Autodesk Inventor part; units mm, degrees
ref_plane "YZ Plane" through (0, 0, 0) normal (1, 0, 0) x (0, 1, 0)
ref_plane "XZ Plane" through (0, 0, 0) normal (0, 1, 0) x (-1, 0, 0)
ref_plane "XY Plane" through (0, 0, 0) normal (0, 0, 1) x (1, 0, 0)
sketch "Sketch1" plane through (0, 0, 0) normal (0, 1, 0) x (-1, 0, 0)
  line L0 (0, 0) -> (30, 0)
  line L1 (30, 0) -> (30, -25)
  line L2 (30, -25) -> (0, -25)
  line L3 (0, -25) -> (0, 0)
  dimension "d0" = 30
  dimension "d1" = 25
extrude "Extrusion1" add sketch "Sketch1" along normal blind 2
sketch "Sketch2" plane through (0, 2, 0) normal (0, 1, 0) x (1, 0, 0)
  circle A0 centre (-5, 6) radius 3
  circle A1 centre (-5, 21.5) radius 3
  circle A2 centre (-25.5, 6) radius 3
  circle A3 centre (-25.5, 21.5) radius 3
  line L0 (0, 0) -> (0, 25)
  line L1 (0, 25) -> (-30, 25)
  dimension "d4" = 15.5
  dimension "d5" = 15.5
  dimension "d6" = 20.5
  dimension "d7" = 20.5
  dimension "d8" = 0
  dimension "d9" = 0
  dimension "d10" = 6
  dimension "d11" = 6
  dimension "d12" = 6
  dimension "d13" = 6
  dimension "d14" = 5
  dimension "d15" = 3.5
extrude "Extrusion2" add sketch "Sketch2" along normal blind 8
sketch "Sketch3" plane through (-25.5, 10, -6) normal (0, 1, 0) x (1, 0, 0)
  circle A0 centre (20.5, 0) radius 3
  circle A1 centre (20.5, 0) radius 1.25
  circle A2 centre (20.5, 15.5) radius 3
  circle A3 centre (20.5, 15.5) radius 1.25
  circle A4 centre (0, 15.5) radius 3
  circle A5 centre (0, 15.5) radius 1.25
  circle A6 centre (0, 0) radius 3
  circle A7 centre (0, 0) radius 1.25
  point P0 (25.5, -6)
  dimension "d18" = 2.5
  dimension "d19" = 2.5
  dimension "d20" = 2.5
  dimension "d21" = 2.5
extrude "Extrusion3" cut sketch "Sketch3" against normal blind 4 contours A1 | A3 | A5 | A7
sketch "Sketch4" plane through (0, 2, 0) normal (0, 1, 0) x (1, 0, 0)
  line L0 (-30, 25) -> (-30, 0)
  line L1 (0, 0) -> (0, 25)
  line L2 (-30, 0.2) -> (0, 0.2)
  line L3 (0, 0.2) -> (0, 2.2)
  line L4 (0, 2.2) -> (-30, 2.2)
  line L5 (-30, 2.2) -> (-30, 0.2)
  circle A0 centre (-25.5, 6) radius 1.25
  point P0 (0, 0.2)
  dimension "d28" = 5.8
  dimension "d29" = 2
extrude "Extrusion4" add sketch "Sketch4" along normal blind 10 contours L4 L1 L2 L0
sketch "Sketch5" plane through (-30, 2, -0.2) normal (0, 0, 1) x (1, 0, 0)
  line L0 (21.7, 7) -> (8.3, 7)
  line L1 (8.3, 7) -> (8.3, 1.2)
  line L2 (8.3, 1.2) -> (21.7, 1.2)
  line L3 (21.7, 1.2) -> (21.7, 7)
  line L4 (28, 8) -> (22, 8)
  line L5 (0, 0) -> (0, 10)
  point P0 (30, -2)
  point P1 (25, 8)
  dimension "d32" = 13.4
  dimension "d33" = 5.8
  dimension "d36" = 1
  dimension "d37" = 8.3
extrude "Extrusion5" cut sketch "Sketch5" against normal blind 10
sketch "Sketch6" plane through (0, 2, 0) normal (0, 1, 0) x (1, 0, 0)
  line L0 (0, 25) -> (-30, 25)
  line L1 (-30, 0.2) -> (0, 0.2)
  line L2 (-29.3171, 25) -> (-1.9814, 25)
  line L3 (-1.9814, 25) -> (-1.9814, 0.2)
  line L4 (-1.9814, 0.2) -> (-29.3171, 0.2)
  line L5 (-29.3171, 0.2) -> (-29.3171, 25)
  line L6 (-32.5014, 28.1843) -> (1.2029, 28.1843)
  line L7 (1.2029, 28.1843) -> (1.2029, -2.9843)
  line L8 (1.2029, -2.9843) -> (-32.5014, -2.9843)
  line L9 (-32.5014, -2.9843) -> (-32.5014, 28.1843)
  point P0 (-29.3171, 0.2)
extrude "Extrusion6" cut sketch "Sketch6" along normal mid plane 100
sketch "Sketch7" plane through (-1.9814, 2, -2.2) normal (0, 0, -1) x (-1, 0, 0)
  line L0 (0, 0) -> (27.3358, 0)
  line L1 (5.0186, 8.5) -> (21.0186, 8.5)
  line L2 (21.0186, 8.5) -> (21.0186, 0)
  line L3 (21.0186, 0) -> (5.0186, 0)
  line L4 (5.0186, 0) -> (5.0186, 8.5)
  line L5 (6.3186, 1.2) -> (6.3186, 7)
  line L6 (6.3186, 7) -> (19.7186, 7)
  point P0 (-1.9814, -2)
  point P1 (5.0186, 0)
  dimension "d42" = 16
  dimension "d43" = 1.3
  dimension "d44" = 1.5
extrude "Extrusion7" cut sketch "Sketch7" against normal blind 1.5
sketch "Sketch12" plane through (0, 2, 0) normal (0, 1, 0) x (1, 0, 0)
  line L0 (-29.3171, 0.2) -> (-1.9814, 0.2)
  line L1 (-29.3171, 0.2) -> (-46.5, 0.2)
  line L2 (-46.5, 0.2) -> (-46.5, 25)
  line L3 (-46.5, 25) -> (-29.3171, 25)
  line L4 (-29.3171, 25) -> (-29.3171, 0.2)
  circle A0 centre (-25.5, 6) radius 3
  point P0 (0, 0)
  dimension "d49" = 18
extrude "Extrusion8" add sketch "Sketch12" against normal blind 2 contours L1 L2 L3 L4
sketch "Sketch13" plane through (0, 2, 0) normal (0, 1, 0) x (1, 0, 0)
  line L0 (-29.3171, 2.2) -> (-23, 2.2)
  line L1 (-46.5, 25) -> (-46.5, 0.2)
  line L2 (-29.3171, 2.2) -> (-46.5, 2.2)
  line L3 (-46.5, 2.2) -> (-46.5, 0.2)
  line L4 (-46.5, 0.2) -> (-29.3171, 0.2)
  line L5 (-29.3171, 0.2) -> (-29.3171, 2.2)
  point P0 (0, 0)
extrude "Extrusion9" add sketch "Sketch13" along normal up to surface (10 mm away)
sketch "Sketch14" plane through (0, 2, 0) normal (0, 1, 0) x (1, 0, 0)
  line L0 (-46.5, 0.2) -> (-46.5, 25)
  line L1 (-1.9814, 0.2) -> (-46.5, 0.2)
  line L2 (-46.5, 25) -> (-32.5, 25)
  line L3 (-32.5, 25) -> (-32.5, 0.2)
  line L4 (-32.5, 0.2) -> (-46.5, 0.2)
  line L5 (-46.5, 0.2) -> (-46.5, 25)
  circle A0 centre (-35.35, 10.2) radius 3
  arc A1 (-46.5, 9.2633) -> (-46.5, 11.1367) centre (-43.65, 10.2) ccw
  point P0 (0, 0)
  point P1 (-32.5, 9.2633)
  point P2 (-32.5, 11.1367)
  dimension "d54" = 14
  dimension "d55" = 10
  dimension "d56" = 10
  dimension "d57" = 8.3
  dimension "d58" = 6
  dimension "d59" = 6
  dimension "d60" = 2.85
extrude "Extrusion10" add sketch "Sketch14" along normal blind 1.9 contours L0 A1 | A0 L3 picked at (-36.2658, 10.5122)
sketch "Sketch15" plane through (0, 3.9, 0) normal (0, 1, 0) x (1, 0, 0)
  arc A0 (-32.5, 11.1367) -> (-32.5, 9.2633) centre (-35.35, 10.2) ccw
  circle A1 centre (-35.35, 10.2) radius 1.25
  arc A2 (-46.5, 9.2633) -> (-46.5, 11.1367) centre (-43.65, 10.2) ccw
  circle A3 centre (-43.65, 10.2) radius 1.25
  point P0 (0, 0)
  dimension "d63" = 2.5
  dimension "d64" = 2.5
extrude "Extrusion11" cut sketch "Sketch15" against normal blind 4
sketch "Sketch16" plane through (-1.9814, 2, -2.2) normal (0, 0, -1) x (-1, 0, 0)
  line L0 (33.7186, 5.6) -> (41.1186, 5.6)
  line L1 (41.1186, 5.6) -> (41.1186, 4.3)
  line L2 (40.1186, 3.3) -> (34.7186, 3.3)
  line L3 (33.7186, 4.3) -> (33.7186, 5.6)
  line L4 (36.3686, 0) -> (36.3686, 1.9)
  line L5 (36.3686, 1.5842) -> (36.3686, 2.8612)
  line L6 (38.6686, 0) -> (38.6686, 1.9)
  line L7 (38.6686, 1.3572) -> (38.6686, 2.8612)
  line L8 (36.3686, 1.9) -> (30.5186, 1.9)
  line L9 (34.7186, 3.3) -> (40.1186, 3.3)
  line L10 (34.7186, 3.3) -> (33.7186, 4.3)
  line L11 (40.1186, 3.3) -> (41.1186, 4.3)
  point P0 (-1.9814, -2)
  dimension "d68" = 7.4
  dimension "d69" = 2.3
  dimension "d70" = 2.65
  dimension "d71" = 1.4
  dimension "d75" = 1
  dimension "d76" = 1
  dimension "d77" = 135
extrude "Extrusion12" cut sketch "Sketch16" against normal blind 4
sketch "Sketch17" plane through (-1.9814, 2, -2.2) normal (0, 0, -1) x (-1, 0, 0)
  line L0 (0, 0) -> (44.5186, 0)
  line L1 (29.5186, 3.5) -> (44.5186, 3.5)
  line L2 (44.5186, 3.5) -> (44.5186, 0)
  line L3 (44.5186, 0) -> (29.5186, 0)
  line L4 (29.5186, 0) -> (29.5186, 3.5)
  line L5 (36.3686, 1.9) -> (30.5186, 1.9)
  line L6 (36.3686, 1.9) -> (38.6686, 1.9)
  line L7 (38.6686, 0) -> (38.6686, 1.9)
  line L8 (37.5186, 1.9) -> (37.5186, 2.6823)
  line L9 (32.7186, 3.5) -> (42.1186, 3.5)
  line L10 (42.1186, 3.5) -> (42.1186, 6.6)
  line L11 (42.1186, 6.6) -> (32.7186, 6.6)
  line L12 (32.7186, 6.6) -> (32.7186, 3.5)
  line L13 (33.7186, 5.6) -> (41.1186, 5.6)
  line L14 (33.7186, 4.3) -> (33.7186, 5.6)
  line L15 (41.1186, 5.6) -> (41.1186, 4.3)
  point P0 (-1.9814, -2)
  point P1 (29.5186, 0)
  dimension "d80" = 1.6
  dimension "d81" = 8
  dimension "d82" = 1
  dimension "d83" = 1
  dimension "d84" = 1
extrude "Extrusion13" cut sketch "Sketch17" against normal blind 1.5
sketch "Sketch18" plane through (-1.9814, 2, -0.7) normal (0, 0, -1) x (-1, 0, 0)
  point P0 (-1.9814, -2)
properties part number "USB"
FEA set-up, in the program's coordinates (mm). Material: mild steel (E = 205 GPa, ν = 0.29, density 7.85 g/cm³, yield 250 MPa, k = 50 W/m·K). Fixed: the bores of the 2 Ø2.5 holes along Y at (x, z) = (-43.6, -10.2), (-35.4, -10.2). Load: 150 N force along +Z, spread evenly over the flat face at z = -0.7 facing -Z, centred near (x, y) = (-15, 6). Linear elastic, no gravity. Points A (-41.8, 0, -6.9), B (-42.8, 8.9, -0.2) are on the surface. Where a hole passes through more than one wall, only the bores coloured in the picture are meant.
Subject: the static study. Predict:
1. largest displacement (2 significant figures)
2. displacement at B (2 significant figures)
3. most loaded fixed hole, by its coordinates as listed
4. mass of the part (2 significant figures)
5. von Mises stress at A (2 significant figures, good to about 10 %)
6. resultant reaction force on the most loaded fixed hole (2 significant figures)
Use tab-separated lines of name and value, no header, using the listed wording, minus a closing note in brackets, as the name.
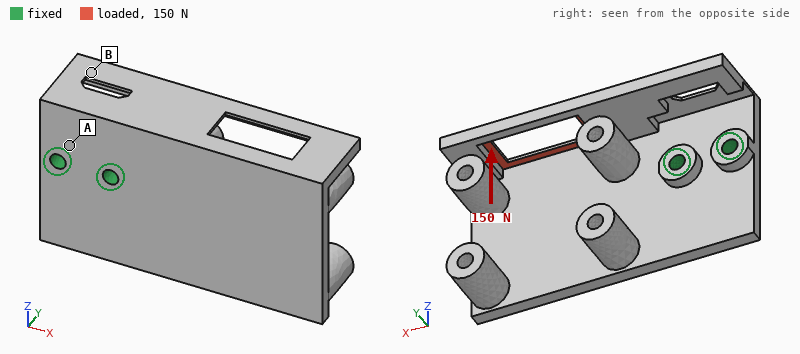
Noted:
largest displacement	64 µm
displacement at B	10 µm
most loaded fixed hole, by its coordinates as listed	(-35.4, -10.2)
mass of the part	28 g
von Mises stress at A	30 MPa
resultant reaction force on the most loaded fixed hole	420 N
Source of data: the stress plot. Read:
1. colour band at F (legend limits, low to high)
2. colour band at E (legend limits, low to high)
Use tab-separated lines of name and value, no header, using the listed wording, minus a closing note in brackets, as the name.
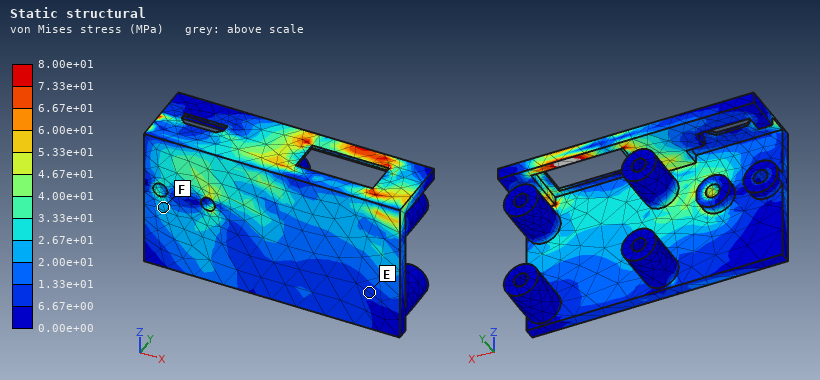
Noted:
colour band at F	2.00e+01 to 2.67e+01 MPa
colour band at E	6.67e+00 to 1.33e+01 MPa
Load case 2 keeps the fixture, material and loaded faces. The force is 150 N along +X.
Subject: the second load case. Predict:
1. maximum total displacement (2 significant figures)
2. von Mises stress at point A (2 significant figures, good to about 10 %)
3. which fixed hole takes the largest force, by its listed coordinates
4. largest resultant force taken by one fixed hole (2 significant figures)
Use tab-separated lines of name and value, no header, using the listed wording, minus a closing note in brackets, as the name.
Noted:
maximum total displacement	35 µm
von Mises stress at point A	24 MPa
which fixed hole takes the largest force, by its listed coordinates	(-35.4, -10.2)
largest resultant force taken by one fixed hole	180 N
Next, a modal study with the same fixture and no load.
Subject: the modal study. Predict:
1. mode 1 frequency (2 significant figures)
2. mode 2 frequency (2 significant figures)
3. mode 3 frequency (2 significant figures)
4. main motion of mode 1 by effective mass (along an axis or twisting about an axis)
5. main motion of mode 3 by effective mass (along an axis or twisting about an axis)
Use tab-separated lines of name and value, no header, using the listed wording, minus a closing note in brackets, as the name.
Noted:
mode 1 frequency	1500 Hz
mode 2 frequency	2500 Hz
mode 3 frequency	5800 Hz
main motion of mode 1 by effective mass	along Y
main motion of mode 3 by effective mass	along Z
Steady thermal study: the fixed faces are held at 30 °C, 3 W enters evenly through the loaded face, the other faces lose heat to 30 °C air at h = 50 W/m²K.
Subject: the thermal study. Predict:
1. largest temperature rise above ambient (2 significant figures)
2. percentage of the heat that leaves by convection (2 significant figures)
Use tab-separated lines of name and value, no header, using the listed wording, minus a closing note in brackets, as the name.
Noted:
largest temperature rise above ambient	36 K
percentage of the heat that leaves by convection	54 %
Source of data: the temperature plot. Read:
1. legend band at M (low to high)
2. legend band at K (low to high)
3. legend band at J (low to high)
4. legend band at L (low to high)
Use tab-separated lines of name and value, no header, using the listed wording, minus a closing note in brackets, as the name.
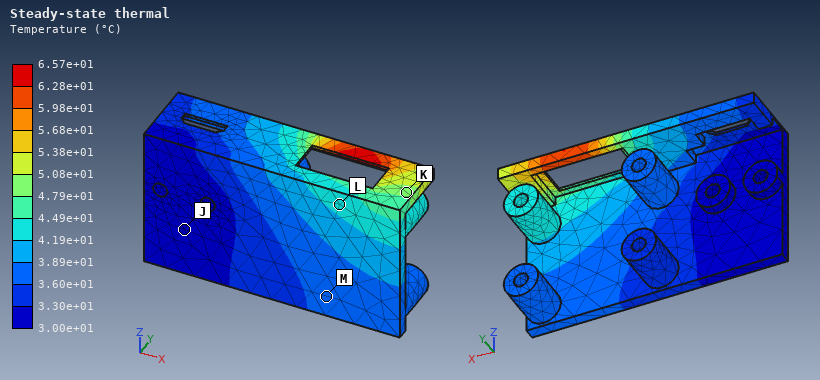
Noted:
legend band at M	3.60e+01 to 3.89e+01 °C
legend band at K	4.79e+01 to 5.08e+01 °C
legend band at J	3.00e+01 to 3.30e+01 °C
legend band at L	4.19e+01 to 4.49e+01 °C
